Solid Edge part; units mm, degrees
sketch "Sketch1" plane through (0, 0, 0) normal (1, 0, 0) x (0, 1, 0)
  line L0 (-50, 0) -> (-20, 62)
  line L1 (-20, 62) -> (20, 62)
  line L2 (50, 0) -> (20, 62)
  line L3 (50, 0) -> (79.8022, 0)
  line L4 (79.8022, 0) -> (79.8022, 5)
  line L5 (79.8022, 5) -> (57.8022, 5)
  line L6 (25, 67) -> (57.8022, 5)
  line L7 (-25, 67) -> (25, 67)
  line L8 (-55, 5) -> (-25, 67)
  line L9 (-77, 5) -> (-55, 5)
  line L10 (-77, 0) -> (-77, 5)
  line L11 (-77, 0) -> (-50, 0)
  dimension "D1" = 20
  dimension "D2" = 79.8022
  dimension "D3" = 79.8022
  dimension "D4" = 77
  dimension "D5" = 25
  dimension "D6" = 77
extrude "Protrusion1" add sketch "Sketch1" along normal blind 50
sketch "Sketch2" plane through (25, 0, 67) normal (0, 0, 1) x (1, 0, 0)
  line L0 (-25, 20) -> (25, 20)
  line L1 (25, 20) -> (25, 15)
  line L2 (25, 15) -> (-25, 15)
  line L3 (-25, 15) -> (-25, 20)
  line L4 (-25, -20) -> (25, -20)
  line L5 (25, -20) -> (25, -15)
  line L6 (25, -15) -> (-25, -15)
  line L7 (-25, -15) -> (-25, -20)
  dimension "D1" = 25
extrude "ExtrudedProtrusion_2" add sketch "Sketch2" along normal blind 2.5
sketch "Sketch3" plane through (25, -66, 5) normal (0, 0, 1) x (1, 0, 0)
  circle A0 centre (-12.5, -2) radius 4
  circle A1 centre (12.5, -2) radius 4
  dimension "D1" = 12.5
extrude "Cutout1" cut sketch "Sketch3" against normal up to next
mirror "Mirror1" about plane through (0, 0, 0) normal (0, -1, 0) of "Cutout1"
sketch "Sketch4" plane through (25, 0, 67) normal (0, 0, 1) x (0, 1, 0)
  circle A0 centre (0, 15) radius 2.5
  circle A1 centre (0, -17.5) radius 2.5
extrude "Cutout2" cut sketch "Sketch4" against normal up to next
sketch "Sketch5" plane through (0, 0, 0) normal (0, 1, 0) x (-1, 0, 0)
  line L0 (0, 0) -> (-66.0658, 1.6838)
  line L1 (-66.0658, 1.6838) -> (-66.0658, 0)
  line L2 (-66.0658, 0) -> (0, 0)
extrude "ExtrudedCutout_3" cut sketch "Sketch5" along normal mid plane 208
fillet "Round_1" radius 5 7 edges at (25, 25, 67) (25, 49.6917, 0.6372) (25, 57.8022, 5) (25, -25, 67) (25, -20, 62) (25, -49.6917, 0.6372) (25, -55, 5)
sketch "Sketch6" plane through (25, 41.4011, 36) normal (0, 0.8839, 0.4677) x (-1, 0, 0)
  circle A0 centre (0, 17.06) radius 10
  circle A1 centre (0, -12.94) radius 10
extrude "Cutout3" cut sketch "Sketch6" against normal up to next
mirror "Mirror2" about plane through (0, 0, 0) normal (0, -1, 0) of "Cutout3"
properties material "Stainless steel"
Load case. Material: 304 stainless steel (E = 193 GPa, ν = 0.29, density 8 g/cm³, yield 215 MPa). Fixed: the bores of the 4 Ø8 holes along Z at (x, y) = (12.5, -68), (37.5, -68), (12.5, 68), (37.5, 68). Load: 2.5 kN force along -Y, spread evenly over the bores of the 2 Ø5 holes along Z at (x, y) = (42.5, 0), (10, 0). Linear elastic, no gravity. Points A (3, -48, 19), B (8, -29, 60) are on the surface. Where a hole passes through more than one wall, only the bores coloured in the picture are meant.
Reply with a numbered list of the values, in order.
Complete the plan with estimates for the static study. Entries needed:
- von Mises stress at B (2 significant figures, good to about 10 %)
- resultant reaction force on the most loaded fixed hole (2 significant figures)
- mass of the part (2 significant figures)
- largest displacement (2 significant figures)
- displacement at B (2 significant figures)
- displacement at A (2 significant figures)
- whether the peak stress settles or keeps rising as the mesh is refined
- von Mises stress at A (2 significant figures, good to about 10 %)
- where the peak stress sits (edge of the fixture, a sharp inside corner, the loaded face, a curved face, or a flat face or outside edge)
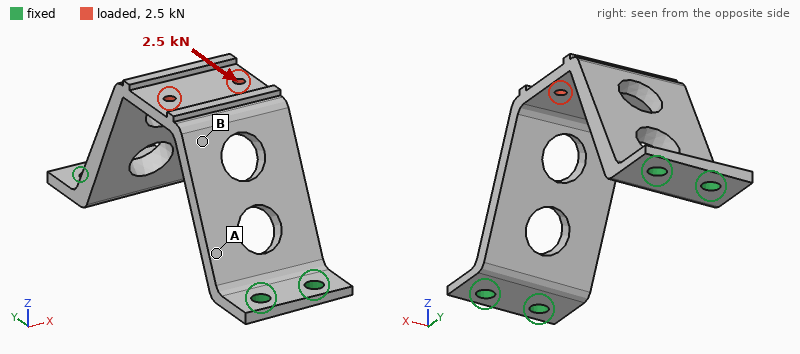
1. 63 MPa
2. 890 N
3. 510 g
4. 0.10 mm
5. 0.097 mm
6. 0.027 mm
7. keeps rising
8. 28 MPa
9. a sharp inside corner
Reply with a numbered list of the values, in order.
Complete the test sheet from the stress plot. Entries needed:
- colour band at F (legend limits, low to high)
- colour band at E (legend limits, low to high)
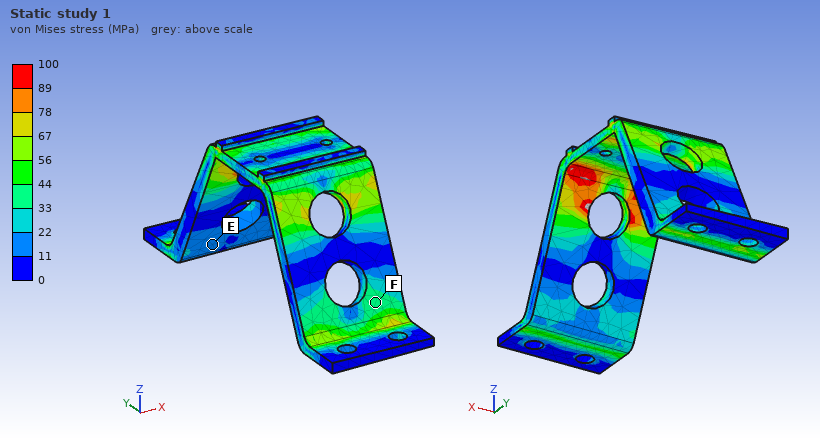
1. 33 to 44 MPa
2. 11 to 22 MPa
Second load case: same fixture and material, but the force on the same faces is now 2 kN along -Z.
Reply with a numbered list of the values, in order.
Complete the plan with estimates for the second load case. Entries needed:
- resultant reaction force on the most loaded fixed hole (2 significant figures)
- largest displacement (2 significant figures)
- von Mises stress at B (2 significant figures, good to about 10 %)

1. 690 N
2. 30 µm
3. 21 MPa
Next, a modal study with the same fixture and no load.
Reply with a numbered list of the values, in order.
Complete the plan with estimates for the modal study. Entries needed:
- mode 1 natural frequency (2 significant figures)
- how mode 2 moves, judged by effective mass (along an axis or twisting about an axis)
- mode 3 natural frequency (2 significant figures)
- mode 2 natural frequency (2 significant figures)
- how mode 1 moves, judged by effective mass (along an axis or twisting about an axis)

1. 1500 Hz
2. along X
3. 2400 Hz
4. 1600 Hz
5. along Y
